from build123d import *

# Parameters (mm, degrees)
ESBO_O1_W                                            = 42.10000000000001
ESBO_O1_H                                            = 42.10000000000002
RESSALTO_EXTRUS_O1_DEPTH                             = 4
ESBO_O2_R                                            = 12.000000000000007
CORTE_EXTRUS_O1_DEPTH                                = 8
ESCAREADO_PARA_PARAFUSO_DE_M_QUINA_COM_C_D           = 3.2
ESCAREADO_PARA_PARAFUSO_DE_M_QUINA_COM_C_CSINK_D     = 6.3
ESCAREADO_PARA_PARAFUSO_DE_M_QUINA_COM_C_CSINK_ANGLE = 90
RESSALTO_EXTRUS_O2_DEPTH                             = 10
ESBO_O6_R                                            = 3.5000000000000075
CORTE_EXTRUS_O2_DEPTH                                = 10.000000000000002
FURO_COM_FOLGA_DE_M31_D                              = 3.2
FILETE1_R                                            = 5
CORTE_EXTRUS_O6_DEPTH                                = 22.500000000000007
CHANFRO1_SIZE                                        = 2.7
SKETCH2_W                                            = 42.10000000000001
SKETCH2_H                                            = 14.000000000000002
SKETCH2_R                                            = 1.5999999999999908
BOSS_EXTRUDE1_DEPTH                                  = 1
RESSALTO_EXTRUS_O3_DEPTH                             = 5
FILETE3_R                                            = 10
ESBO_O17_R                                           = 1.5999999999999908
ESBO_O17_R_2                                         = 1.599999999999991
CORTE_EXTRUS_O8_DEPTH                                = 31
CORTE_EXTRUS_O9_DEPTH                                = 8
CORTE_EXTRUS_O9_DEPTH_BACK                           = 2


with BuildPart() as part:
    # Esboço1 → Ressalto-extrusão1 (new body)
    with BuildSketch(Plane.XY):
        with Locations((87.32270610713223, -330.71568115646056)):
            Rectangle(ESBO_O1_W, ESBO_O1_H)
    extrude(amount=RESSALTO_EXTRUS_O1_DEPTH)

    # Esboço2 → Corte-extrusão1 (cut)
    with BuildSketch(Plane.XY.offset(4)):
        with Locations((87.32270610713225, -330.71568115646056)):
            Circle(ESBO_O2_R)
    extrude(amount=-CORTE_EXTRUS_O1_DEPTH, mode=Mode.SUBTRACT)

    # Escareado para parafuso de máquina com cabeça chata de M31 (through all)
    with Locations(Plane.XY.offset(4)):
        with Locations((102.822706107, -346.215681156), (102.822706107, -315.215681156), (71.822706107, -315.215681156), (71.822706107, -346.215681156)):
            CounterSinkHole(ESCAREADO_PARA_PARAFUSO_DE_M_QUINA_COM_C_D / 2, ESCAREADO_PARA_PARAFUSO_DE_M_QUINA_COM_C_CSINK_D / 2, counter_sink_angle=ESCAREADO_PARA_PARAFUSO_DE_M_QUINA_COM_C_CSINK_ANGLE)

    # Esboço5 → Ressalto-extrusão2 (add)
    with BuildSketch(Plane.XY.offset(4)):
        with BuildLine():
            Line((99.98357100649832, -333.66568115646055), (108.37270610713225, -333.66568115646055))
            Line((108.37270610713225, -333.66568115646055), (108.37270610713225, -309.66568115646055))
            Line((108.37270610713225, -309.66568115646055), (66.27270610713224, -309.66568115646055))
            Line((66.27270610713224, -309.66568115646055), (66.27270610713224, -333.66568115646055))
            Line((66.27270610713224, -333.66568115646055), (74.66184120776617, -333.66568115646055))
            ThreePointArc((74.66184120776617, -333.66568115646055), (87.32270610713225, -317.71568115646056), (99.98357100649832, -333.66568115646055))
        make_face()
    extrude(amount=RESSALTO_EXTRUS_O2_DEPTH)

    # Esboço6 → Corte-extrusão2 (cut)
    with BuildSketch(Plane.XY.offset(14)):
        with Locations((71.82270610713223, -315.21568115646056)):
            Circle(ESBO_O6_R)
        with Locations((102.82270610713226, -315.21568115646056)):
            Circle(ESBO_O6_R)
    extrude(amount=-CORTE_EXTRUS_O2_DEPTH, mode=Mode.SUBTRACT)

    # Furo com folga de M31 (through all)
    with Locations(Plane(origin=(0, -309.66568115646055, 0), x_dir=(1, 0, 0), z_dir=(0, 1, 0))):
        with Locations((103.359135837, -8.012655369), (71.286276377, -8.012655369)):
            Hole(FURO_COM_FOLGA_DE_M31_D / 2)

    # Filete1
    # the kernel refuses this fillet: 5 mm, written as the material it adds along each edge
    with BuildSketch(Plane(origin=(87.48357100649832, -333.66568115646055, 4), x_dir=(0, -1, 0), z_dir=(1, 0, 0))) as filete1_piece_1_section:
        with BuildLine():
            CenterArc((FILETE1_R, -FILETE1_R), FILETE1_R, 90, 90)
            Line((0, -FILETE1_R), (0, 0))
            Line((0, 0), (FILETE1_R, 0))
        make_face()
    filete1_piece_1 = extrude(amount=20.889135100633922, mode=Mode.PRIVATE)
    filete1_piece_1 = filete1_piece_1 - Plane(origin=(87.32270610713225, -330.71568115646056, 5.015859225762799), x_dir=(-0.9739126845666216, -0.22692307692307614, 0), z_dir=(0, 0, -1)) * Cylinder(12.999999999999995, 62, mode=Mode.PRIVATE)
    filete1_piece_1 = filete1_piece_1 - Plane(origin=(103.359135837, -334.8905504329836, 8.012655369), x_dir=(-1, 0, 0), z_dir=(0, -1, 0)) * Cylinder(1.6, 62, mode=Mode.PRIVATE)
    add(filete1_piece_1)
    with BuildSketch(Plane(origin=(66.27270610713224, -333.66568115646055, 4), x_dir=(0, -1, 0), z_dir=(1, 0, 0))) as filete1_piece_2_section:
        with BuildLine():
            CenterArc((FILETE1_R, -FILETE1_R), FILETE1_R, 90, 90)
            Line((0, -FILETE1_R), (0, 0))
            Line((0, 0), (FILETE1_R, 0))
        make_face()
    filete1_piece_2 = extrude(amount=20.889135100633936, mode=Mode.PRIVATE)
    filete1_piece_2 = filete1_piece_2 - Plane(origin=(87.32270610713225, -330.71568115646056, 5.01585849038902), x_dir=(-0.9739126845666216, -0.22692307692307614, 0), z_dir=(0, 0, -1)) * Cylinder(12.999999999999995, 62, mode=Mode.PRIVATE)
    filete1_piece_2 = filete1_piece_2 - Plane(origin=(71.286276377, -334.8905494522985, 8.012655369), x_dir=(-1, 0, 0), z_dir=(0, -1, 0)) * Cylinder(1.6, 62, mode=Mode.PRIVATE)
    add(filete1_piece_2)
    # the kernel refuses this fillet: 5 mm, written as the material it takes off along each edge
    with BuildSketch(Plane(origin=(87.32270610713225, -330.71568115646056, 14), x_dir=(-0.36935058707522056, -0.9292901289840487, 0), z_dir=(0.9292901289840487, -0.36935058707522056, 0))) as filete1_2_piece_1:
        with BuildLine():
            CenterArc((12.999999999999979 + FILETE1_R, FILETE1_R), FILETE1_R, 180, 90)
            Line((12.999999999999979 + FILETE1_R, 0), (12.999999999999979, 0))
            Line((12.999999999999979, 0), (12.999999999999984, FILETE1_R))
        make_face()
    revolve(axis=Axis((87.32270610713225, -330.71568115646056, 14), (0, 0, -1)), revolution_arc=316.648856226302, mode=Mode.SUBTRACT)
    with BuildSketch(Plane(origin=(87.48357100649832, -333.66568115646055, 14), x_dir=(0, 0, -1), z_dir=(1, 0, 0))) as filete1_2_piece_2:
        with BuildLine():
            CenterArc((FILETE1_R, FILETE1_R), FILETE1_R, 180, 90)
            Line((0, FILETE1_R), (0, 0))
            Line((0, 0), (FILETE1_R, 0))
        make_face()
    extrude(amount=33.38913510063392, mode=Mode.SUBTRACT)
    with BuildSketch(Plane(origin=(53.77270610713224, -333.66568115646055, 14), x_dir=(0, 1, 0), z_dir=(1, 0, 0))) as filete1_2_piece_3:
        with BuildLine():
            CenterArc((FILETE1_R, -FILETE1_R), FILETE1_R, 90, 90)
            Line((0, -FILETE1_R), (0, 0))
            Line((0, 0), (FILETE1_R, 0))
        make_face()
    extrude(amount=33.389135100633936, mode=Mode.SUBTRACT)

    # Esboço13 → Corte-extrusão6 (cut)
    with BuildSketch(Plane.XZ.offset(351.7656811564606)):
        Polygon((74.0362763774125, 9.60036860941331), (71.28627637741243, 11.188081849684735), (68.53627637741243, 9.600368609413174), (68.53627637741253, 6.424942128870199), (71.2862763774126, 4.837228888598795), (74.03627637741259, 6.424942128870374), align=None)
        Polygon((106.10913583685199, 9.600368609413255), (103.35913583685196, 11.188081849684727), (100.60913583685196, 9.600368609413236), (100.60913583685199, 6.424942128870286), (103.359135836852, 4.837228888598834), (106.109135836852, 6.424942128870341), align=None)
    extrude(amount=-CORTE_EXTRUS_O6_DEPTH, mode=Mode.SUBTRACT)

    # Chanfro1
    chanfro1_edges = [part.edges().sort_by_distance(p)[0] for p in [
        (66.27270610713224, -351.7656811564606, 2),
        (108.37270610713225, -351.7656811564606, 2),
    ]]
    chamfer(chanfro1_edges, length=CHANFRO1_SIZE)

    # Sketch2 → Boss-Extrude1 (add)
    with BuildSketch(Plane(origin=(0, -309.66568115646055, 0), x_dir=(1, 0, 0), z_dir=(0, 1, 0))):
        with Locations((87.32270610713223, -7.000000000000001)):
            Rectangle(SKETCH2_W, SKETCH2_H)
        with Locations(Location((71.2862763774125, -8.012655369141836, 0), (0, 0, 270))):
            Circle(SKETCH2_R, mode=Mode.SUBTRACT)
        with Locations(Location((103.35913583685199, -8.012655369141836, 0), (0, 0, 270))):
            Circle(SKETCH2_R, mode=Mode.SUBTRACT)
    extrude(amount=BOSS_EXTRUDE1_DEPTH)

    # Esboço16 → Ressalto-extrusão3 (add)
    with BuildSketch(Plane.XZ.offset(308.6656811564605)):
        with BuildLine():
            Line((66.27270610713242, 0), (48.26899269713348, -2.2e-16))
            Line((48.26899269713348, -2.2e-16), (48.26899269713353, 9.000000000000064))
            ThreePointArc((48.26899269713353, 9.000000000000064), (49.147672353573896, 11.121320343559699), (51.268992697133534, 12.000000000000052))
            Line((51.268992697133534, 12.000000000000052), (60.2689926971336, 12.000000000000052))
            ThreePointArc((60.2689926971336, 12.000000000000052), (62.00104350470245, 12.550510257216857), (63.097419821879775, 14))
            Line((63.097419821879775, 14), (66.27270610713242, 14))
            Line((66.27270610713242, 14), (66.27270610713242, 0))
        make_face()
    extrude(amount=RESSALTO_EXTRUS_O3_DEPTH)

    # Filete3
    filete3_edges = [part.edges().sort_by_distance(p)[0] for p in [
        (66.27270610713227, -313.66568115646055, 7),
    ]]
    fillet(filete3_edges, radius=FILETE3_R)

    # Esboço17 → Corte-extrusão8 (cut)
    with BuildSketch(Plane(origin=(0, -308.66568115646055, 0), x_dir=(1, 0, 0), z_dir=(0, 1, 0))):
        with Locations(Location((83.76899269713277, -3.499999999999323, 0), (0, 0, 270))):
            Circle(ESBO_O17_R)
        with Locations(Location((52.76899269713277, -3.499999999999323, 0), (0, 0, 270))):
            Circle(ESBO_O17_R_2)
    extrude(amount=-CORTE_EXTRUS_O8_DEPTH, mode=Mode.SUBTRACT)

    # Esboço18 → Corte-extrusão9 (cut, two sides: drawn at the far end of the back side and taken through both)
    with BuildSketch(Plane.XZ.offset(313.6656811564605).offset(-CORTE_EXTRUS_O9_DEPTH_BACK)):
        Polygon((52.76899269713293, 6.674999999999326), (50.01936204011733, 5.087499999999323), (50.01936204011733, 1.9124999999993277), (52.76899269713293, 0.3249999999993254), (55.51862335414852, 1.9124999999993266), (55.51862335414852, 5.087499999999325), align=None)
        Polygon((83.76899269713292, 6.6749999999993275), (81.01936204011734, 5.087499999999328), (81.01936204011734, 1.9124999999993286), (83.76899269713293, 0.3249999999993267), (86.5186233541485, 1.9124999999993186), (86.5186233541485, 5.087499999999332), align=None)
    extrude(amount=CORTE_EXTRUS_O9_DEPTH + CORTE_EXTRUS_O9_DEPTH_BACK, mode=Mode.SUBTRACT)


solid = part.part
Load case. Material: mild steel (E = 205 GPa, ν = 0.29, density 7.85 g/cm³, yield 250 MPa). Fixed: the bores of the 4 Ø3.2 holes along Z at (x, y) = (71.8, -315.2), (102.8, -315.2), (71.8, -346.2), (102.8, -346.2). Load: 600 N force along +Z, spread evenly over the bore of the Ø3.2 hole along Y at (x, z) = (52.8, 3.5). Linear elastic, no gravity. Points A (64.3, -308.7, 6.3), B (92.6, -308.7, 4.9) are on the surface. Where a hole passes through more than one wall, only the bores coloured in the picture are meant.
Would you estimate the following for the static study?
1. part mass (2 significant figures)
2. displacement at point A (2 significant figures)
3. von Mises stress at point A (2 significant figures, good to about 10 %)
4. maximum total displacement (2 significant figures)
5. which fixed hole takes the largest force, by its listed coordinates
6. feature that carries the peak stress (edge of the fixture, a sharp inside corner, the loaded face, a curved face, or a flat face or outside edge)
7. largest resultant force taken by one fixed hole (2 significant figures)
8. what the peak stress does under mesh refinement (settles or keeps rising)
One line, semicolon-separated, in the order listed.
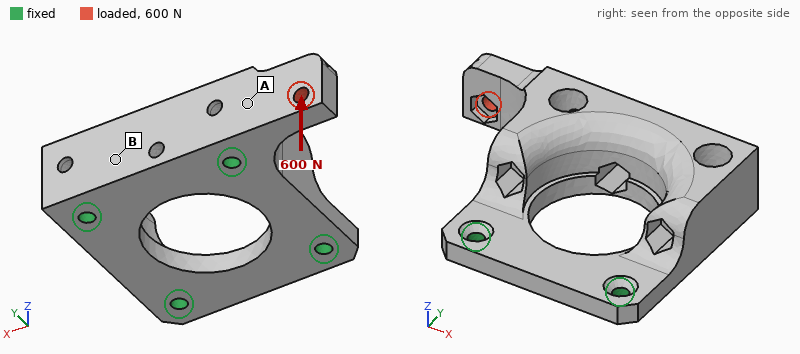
94 g; 5.0 µm; 12 MPa; 17 µm; (71.8, -315.2); edge of the fixture; 1.1 kN; keeps rising
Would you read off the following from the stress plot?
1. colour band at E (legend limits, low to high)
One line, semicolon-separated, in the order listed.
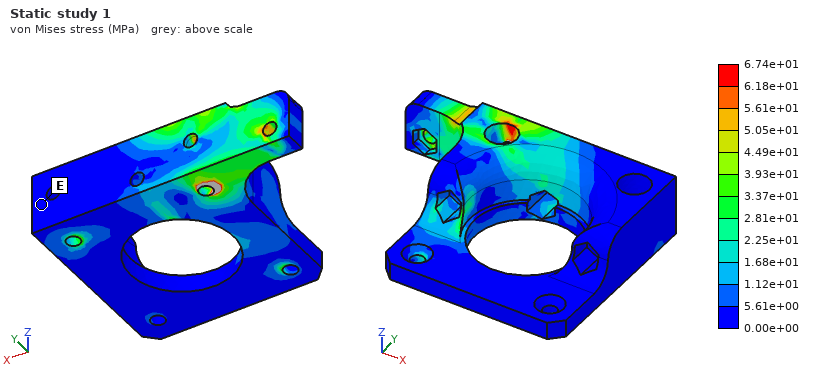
0.00e+00 to 5.61e+00 MPa
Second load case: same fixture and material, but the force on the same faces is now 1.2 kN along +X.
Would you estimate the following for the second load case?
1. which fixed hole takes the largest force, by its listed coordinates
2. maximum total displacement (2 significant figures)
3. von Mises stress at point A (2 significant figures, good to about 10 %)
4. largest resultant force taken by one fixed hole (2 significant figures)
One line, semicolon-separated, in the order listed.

(71.8, -315.2); 14 µm; 32 MPa; 980 N
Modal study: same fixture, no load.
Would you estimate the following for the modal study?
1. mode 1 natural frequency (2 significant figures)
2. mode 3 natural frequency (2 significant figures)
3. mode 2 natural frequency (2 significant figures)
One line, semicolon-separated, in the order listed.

13 kHz; 14 kHz; 13 kHz
